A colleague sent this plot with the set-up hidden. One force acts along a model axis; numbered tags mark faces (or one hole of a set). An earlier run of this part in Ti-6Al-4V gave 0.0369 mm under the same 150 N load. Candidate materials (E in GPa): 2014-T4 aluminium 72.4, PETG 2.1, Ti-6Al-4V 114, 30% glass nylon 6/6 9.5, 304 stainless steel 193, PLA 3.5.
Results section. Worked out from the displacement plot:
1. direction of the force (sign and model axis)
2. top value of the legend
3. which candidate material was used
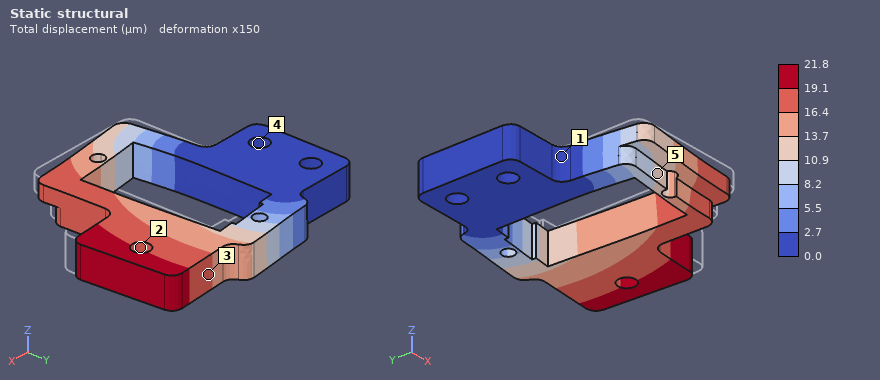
+Y
21.8 µm
304 stainless steel
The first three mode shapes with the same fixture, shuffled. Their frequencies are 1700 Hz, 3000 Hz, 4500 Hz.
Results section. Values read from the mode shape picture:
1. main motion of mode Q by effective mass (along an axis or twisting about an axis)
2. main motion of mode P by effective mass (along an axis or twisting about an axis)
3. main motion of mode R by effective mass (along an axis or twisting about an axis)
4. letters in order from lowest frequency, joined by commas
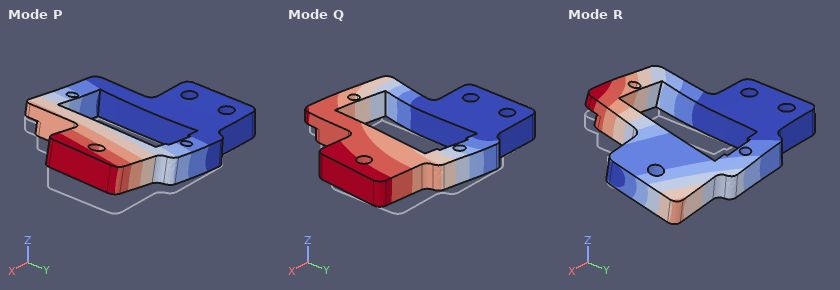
along Y
along Z
twisting about X
P, Q, R
